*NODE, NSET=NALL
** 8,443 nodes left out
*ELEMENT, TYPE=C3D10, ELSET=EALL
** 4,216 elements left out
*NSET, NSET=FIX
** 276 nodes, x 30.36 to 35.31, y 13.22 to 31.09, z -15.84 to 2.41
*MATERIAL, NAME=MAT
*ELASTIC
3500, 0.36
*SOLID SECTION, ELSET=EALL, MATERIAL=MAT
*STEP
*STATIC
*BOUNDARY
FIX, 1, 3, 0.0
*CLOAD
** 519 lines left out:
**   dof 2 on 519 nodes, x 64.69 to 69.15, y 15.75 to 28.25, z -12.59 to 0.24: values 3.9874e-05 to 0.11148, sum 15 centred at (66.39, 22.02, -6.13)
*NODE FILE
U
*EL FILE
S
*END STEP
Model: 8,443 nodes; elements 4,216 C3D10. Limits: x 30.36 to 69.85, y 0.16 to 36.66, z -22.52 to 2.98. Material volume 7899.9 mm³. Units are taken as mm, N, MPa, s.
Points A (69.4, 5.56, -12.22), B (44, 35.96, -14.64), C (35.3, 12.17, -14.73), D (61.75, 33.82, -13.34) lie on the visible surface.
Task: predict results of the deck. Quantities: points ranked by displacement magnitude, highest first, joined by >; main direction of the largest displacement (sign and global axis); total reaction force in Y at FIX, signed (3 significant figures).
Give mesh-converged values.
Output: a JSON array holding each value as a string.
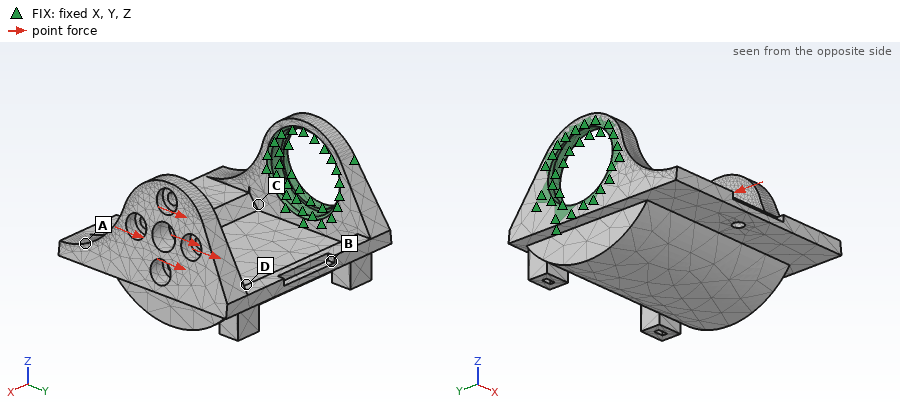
["A > D > B > C", "+Y", "-15.0 N"]
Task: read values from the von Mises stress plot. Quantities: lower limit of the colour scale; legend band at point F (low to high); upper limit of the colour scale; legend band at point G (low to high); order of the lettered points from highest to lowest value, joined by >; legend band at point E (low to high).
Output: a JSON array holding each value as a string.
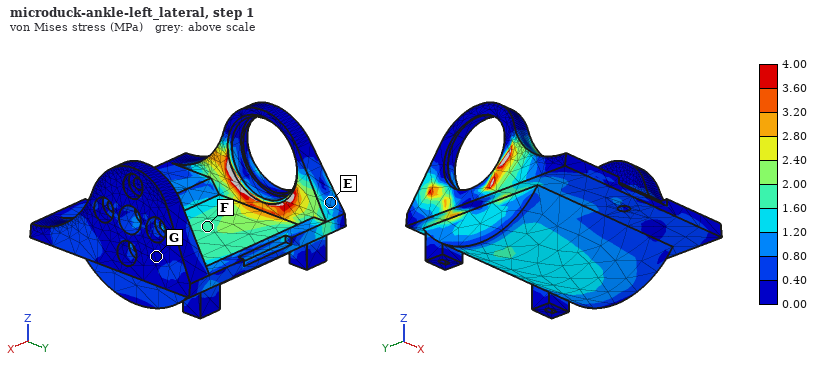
["0.00 MPa", "1.60 to 2.00 MPa", "4.00 MPa", "0.00 to 0.40 MPa", "F > E > G", "0.80 to 1.20 MPa"]
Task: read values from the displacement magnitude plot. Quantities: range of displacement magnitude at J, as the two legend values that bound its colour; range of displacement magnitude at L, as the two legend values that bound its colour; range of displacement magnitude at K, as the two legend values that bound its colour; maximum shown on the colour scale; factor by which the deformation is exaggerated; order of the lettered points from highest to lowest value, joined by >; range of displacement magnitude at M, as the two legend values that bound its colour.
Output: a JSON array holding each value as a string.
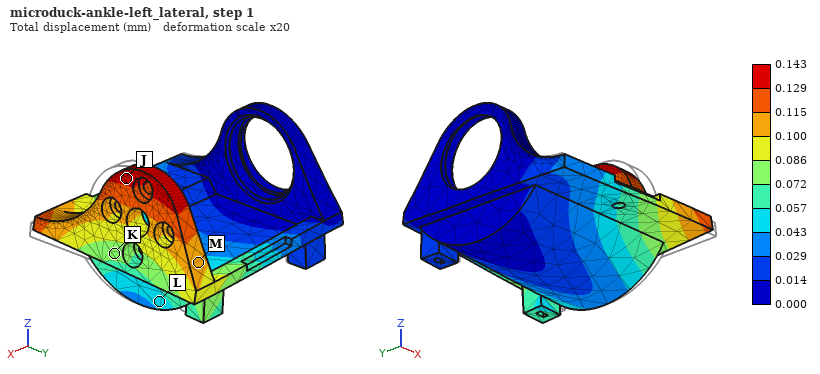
["0.129 to 0.143 mm", "0.043 to 0.057 mm", "0.072 to 0.086 mm", "0.143 mm", "20", "J > M > K > L", "0.100 to 0.115 mm"]
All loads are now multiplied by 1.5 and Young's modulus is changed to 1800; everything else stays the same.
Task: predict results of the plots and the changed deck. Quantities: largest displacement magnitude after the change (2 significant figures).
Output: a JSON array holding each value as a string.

["0.42 mm"]
